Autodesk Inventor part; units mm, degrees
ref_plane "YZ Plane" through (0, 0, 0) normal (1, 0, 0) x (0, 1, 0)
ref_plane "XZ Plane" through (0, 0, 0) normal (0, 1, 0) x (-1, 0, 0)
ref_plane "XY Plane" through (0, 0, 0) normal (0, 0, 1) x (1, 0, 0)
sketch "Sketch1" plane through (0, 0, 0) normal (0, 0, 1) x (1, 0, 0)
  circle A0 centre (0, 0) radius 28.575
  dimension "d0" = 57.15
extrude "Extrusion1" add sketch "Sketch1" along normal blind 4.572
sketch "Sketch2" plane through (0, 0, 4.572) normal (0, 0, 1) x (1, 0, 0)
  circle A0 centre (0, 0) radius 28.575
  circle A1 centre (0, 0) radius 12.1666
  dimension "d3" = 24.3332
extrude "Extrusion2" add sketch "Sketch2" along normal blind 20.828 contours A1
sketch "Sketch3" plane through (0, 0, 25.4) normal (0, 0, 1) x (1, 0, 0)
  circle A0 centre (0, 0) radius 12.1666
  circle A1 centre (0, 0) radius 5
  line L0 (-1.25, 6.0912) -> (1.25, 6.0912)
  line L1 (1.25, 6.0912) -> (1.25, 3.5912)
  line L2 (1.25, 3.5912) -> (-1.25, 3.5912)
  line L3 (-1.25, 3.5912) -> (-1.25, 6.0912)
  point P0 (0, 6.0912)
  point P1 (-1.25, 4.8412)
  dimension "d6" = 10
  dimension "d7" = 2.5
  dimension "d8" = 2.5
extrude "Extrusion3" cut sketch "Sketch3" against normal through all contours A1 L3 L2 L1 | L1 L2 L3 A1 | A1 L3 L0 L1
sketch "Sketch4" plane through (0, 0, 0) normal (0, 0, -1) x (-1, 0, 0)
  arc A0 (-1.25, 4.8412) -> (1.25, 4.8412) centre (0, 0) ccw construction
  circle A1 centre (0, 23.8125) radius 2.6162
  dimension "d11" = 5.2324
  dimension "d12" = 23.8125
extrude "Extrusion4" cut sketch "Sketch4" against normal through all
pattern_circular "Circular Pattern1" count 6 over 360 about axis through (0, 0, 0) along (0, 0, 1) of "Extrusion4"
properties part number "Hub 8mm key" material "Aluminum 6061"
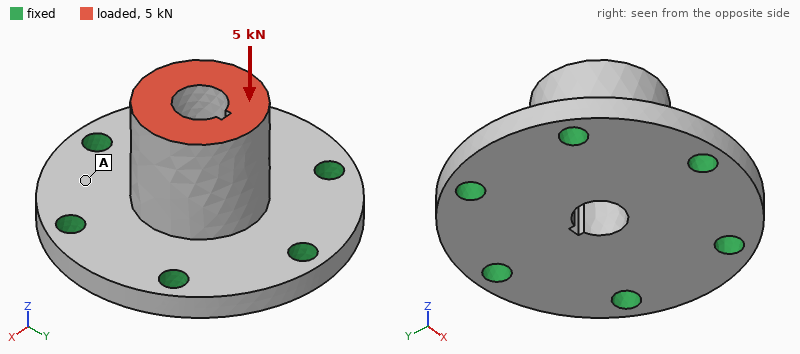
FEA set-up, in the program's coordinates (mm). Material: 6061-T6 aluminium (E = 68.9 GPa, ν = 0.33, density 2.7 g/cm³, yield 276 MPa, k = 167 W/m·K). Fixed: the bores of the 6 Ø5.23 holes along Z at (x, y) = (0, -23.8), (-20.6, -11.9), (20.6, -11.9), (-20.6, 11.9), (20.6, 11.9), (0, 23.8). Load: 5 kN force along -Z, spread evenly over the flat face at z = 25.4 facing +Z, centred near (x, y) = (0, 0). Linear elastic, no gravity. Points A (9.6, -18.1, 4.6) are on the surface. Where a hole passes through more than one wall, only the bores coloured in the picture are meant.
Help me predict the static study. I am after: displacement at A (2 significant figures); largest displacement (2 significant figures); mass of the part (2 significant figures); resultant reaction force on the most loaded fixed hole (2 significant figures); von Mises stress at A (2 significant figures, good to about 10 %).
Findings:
6.1 µm
28 µm
51 g
920 N
22 MPa
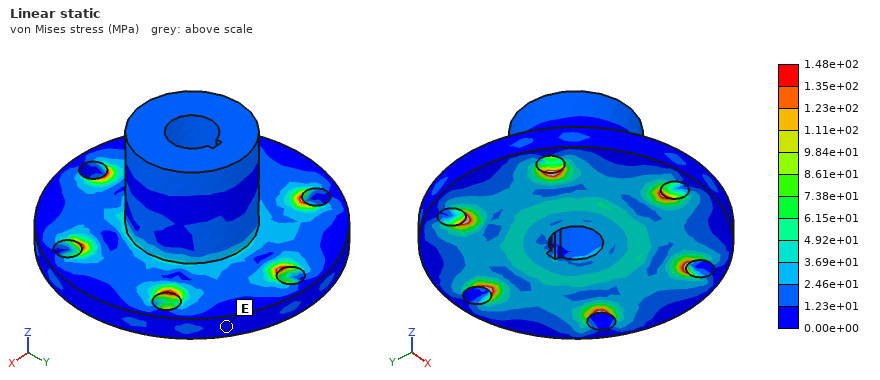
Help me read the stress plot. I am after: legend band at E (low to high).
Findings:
0.00e+00 to 1.23e+01 MPa
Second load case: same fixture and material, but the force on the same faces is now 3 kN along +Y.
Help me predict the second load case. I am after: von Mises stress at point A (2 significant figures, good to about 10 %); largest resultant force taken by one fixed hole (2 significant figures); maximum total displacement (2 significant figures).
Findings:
24 MPa
1.5 kN
72 µm
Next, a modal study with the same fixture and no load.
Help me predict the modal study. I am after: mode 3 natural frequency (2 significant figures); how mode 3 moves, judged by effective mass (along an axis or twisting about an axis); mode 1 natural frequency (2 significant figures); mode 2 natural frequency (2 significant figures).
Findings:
13 kHz
along Z
11 kHz
11 kHz
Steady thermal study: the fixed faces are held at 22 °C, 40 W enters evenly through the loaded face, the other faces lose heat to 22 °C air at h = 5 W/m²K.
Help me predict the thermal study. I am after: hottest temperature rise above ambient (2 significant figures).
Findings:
21 K
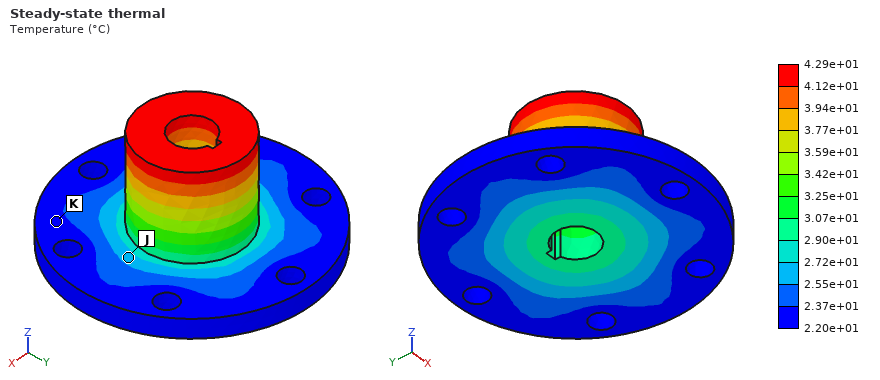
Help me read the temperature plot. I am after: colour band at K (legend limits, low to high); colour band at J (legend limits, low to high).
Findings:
2.20e+01 to 2.37e+01 °C
2.55e+01 to 2.72e+01 °C
